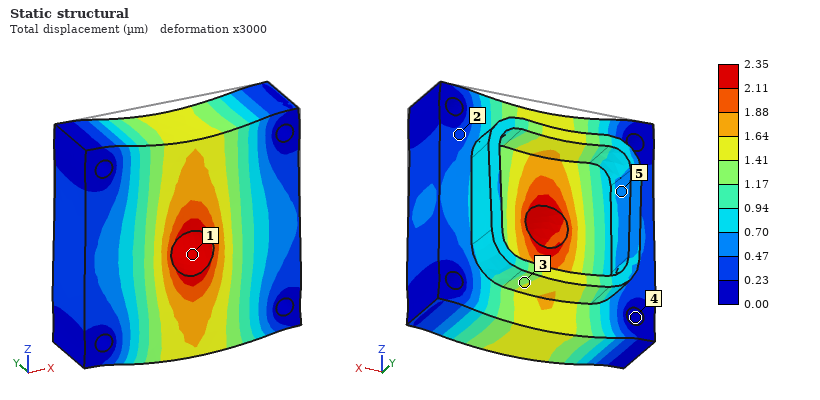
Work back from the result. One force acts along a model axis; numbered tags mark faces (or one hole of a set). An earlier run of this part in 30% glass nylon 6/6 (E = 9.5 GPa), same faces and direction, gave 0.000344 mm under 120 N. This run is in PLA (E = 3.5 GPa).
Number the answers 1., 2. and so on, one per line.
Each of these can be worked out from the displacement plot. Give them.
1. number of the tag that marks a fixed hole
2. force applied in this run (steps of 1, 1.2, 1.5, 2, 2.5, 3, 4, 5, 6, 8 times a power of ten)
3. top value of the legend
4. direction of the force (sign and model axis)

1. 4
2. 300 N
3. 2.35 µm
4. -Z
